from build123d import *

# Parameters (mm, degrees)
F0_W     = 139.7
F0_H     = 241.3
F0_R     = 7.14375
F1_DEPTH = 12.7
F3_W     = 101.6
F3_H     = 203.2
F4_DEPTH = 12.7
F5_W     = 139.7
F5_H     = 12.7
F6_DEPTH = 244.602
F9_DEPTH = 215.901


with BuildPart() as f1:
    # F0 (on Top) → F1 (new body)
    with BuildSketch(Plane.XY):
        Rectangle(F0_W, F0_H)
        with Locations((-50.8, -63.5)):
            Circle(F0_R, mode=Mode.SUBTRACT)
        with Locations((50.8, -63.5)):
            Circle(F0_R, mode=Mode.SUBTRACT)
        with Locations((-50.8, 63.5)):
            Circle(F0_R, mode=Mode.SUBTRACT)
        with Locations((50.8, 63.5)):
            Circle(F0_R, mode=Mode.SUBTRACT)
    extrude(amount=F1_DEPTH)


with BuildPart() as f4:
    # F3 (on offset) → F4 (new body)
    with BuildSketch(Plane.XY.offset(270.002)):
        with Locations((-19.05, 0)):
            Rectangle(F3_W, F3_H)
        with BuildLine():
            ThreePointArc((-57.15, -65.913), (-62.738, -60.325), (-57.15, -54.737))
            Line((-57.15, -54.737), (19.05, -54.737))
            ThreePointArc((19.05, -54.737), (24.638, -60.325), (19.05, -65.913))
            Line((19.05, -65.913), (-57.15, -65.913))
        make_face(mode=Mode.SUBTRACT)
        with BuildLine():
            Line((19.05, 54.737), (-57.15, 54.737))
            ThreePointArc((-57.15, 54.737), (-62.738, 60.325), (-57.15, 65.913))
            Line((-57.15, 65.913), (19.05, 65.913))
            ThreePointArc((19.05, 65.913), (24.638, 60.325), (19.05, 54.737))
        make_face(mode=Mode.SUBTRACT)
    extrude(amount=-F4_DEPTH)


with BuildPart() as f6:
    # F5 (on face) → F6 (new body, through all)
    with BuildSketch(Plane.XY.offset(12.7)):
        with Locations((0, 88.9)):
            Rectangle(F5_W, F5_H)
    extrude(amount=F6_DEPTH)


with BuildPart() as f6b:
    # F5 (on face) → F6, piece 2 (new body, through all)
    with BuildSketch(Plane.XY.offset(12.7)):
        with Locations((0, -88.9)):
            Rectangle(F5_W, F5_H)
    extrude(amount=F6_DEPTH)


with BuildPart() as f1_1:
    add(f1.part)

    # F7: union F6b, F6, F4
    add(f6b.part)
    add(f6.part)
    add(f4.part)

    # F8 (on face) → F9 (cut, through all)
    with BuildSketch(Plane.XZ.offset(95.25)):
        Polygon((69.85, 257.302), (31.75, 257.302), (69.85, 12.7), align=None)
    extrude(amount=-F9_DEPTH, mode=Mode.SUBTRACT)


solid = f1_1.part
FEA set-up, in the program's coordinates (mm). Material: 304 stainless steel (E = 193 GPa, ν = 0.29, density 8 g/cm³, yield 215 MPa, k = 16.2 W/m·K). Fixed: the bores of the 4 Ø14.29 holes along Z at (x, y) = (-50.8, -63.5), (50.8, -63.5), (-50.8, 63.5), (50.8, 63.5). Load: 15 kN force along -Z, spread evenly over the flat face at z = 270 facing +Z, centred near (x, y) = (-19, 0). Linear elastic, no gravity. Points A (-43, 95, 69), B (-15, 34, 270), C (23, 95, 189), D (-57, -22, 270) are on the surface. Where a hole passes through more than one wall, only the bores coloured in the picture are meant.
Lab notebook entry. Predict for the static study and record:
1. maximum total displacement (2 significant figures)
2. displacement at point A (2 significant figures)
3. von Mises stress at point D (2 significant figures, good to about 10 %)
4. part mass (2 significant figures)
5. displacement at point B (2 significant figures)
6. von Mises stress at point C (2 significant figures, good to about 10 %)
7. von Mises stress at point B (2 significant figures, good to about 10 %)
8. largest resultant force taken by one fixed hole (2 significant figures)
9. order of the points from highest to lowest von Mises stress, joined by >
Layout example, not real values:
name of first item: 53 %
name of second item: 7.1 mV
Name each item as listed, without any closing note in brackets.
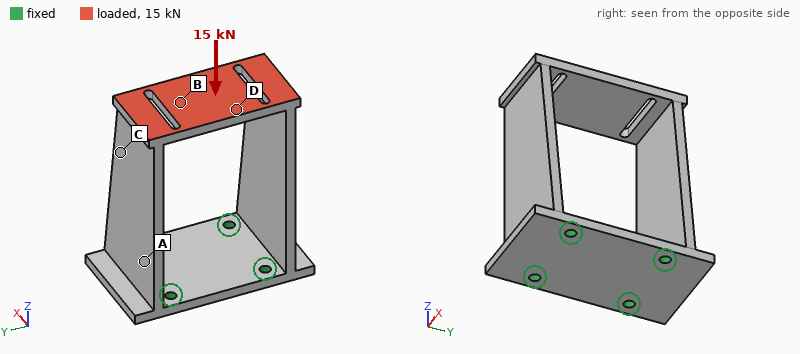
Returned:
maximum total displacement: 0.22 mm
displacement at point A: 0.061 mm
von Mises stress at point D: 59 MPa
part mass: 11 kg
displacement at point B: 0.19 mm
von Mises stress at point C: 21 MPa
von Mises stress at point B: 30 MPa
largest resultant force taken by one fixed hole: 5.1 kN
order of the points from highest to lowest von Mises stress, joined by >: D > B > C > A
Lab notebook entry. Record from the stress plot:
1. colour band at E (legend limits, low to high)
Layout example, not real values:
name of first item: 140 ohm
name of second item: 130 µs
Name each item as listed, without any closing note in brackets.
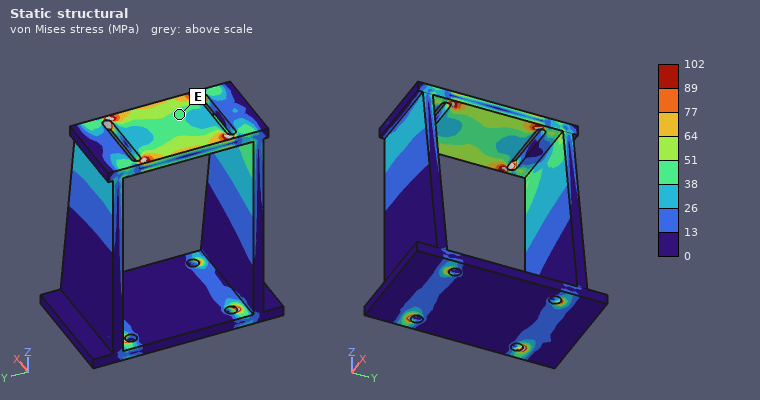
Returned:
colour band at E: 38 to 51 MPa
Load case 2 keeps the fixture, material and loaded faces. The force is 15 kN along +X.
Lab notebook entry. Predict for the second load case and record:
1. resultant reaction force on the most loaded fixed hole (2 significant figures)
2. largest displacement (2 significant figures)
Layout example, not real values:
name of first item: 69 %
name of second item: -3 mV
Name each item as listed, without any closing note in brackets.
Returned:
resultant reaction force on the most loaded fixed hole: 19 kN
largest displacement: 0.35 mm
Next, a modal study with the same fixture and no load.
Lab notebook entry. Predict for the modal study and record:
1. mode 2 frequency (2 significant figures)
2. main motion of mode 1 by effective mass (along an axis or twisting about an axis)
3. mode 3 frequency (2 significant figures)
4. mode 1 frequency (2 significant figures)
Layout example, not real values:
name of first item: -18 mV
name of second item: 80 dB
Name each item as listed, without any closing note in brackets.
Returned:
mode 2 frequency: 590 Hz
main motion of mode 1 by effective mass: along Y
mode 3 frequency: 610 Hz
mode 1 frequency: 130 Hz
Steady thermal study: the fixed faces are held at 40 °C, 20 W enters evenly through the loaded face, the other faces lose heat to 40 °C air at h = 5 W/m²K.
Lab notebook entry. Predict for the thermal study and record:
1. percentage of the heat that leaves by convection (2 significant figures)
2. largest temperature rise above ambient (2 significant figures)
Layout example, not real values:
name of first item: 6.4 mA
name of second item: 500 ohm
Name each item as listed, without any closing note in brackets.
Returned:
percentage of the heat that leaves by convection: 84 %
largest temperature rise above ambient: 70 K
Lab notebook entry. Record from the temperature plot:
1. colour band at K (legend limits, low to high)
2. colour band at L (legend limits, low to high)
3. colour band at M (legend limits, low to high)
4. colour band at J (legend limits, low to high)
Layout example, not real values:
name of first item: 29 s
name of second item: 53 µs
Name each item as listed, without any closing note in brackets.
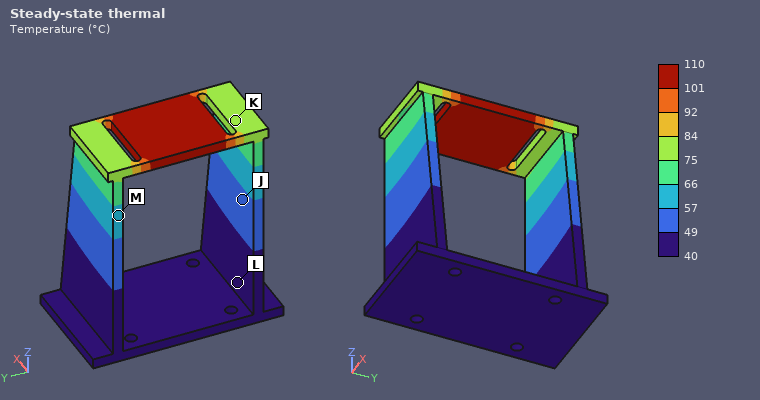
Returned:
colour band at K: 75 to 84 °C
colour band at L: 40 to 49 °C
colour band at M: 57 to 66 °C
colour band at J: 49 to 57 °C
